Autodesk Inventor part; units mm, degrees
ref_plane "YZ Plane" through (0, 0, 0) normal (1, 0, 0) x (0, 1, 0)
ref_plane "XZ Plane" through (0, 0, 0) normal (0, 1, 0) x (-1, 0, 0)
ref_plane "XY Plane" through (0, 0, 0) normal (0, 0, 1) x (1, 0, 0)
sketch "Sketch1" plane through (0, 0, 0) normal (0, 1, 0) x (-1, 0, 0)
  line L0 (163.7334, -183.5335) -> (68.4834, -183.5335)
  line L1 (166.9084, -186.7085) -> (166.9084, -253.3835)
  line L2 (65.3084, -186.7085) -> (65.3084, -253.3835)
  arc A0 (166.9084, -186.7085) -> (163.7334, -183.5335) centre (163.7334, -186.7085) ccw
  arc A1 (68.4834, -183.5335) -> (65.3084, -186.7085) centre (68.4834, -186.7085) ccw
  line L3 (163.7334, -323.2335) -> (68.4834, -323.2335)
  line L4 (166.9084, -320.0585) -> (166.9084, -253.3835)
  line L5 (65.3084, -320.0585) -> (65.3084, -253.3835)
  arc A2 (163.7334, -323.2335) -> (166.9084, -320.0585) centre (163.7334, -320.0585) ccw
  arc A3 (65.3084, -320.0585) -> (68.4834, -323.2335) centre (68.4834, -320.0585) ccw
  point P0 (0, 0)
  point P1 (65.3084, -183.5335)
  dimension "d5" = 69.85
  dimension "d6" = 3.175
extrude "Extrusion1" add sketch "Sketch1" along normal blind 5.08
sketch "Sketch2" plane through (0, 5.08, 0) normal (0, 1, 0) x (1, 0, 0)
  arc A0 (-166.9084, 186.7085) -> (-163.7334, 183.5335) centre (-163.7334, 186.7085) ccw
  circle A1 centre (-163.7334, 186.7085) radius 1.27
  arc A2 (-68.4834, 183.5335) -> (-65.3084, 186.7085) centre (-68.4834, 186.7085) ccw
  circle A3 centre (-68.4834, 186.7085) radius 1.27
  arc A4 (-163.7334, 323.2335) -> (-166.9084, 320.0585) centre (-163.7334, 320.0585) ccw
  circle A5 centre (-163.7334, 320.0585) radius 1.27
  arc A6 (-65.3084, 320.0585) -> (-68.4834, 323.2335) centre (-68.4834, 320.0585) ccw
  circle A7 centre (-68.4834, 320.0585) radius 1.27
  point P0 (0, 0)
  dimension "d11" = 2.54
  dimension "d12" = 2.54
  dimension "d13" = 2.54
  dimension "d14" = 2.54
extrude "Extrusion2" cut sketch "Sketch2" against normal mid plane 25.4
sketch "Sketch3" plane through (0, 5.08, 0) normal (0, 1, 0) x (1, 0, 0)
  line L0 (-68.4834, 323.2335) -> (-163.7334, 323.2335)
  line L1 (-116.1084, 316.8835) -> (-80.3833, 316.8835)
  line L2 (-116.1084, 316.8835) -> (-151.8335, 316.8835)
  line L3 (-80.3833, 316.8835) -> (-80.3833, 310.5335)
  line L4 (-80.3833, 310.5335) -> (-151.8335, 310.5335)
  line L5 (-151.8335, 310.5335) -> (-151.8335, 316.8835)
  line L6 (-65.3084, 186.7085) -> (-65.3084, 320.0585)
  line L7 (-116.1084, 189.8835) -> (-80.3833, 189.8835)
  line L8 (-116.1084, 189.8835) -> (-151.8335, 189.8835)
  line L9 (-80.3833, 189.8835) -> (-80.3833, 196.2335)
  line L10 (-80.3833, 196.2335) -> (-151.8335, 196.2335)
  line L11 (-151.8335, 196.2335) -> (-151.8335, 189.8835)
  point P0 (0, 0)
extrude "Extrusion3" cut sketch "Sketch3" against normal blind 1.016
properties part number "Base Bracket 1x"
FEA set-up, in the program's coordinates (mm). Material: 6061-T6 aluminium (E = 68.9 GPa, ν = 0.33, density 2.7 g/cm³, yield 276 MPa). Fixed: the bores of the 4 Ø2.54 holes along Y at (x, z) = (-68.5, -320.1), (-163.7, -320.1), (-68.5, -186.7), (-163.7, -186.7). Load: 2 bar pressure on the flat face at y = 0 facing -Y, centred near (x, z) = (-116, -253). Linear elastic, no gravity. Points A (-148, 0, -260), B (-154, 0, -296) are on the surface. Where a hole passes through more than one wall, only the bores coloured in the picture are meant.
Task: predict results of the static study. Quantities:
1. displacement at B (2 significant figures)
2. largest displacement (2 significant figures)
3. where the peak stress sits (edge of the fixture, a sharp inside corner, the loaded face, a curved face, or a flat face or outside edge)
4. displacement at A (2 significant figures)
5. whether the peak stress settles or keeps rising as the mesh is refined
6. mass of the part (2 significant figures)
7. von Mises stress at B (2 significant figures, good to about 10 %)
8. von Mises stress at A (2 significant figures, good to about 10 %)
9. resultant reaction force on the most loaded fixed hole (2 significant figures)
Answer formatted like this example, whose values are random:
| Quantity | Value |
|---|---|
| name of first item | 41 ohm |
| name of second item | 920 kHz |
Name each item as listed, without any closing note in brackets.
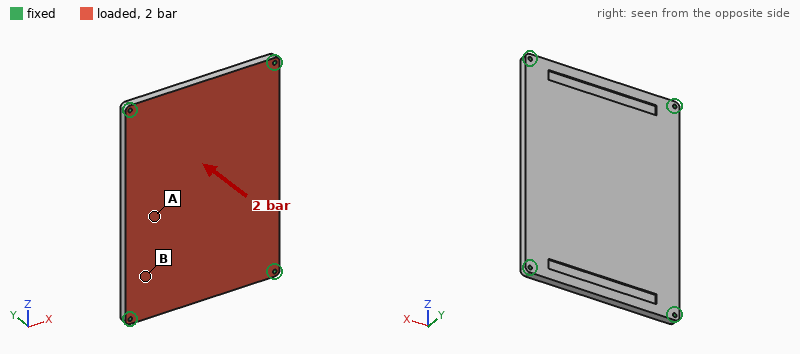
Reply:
| Quantity | Value |
|---|---|
| displacement at B | 0.24 mm |
| largest displacement | 0.52 mm |
| where the peak stress sits | edge of the fixture |
| displacement at A | 0.48 mm |
| whether the peak stress settles or keeps rising as the mesh is refined | keeps rising |
| mass of the part | 190 g |
| von Mises stress at B | 22 MPa |
| von Mises stress at A | 50 MPa |
| resultant reaction force on the most loaded fixed hole | 710 N |
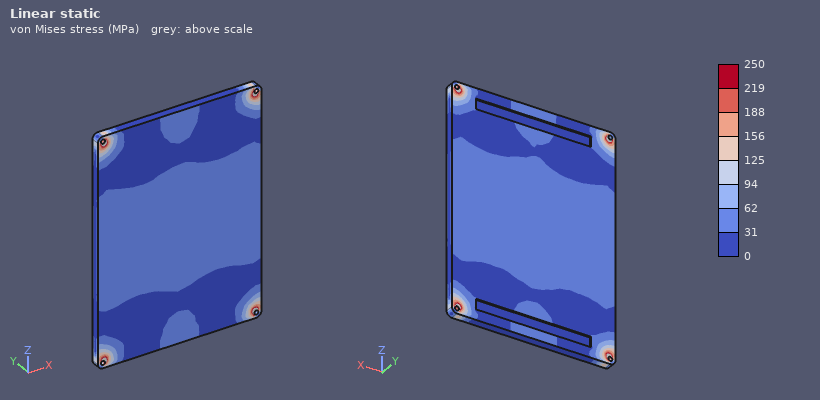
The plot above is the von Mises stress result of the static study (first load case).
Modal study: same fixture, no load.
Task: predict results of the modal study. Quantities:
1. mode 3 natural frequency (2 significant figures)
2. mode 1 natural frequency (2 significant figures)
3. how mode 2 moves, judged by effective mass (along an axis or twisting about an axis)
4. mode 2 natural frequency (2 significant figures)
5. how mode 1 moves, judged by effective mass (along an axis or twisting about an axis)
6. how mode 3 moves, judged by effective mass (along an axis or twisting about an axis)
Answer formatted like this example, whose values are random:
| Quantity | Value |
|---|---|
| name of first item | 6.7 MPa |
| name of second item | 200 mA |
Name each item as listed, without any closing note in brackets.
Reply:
| Quantity | Value |
|---|---|
| mode 3 natural frequency | 2300 Hz |
| mode 1 natural frequency | 970 Hz |
| how mode 2 moves, judged by effective mass | twisting about Z |
| mode 2 natural frequency | 1700 Hz |
| how mode 1 moves, judged by effective mass | along Y |
| how mode 3 moves, judged by effective mass | twisting about X |
